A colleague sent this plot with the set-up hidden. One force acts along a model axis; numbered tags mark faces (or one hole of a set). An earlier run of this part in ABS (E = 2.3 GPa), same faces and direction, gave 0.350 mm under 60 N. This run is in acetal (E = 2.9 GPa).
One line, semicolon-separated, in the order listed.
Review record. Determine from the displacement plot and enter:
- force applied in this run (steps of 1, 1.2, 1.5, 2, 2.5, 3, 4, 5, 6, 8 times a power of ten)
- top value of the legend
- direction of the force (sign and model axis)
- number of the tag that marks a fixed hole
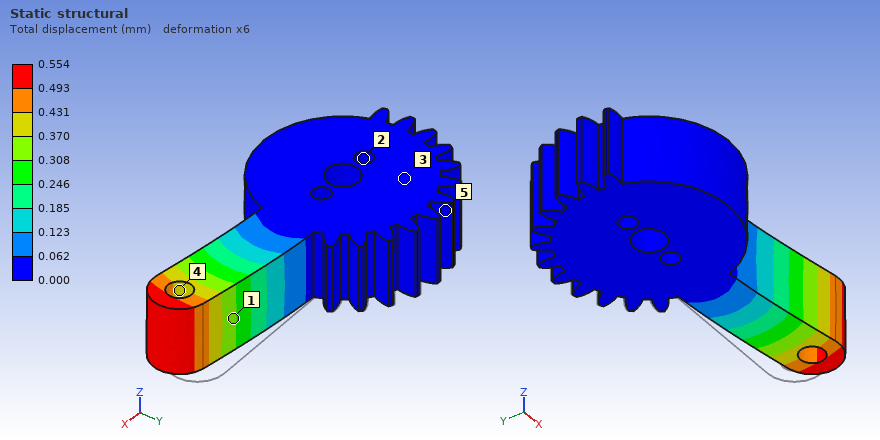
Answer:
120 N; 0.554 mm; -Y; 2
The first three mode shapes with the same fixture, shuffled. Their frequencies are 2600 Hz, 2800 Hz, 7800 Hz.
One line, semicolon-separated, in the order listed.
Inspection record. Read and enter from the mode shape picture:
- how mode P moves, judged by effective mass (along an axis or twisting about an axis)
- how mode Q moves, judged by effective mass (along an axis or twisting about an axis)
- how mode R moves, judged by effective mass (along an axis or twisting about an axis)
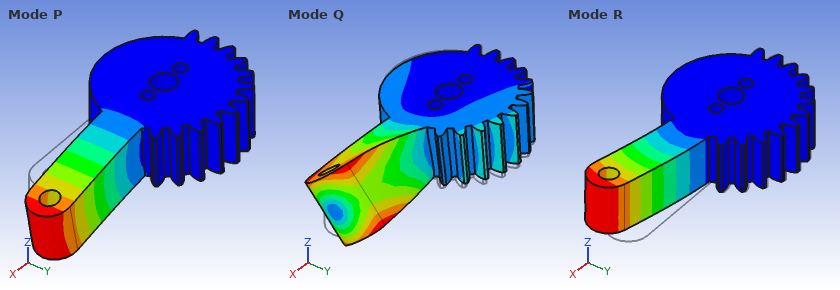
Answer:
along Z; twisting about X; along Y
